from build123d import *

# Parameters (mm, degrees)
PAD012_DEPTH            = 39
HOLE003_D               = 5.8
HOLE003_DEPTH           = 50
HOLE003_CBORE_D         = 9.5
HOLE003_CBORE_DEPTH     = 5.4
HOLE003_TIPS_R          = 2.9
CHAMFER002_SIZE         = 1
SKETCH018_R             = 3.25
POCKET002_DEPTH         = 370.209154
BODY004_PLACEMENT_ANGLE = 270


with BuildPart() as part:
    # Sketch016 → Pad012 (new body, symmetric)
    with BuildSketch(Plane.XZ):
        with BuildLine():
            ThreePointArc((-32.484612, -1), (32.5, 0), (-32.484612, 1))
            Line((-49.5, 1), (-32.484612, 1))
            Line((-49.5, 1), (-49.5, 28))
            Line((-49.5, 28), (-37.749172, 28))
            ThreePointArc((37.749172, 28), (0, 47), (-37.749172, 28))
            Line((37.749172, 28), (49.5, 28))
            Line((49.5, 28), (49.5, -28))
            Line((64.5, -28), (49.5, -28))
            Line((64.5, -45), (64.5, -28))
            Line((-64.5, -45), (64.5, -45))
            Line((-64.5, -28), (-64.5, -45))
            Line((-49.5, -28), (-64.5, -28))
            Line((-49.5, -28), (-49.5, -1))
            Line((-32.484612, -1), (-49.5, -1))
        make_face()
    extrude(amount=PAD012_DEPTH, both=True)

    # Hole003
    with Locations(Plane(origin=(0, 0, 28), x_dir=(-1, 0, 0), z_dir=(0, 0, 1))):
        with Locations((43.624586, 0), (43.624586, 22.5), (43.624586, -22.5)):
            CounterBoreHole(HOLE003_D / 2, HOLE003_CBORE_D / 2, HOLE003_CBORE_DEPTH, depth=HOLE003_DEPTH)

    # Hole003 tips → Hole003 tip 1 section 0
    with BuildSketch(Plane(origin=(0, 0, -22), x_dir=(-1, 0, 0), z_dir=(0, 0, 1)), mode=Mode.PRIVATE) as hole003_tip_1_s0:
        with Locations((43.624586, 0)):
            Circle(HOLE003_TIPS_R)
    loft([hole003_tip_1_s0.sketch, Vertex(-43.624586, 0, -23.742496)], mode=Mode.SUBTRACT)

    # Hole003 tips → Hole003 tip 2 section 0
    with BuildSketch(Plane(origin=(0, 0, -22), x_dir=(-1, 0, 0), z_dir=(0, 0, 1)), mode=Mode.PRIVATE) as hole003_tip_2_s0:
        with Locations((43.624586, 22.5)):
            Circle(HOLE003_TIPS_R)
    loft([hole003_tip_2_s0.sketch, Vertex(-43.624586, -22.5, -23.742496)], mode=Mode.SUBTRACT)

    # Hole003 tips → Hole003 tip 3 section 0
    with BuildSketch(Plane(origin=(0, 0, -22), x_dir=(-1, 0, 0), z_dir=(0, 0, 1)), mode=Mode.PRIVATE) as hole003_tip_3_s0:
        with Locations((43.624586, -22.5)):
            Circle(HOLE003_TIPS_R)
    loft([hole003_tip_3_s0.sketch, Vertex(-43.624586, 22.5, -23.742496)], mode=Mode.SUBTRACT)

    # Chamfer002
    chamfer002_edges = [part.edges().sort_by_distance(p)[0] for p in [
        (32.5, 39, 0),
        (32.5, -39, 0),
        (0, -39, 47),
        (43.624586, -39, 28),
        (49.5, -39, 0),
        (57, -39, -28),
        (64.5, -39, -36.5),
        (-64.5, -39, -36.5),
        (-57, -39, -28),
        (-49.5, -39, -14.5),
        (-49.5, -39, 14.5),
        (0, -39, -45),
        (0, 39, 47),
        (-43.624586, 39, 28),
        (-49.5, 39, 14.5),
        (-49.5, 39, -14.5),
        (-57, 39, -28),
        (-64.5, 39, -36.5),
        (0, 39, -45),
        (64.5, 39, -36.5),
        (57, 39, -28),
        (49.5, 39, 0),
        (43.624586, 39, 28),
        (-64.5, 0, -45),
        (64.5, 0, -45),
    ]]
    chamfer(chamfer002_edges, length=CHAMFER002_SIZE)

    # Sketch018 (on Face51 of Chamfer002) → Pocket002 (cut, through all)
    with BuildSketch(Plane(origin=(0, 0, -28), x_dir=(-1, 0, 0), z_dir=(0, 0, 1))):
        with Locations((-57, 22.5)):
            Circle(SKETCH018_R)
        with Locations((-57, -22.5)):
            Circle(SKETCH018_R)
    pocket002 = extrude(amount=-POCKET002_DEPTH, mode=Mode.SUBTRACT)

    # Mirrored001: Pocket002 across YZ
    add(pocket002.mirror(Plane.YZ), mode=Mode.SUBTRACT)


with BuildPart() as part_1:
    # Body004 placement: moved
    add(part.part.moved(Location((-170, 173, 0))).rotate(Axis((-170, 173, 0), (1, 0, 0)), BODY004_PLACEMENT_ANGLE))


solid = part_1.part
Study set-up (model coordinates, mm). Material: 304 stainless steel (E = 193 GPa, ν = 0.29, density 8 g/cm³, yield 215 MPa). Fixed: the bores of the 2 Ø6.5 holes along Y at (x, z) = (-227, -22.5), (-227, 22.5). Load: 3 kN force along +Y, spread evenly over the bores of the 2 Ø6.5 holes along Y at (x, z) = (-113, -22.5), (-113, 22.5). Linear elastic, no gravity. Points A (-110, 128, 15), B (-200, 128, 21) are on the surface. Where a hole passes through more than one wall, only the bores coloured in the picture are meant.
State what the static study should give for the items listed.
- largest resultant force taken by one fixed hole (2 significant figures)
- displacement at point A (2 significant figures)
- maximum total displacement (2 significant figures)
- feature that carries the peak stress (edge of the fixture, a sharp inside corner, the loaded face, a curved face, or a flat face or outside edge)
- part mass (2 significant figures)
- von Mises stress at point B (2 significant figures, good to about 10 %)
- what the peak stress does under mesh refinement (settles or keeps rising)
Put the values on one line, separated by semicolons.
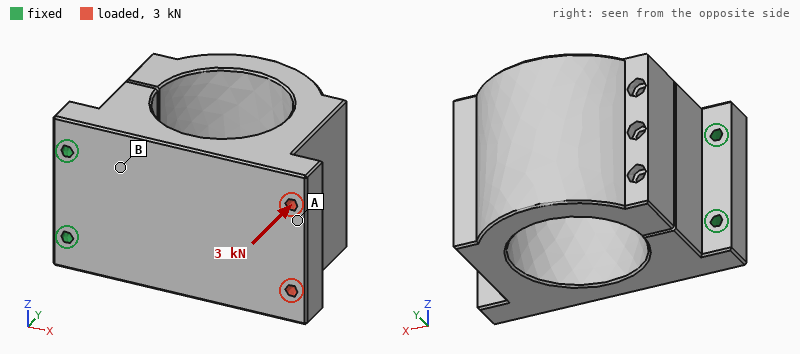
1.6 kN; 0.28 mm; 0.33 mm; edge of the fixture; 3.3 kg; 42 MPa; keeps rising
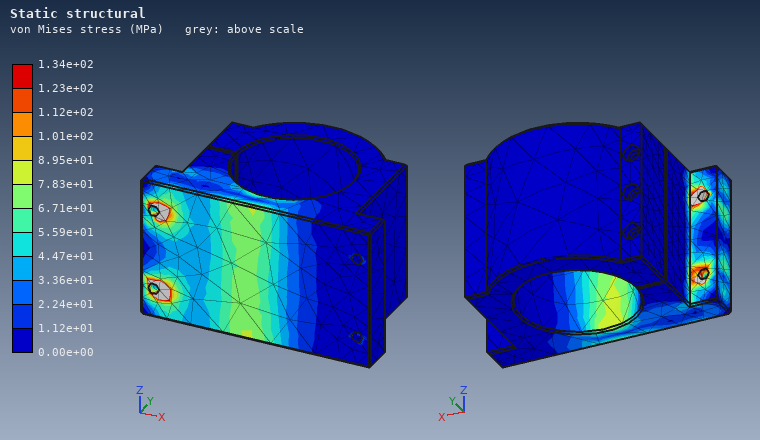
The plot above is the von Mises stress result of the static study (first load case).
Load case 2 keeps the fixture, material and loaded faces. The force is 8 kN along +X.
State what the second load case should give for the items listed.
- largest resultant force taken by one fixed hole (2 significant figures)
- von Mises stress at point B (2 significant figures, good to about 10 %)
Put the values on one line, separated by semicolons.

4.0 kN; 7.9 MPa
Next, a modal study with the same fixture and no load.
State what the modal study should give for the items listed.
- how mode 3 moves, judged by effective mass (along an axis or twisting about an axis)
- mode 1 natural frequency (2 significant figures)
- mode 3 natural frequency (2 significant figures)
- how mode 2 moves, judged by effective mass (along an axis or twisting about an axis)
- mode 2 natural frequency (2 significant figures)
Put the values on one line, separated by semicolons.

along Y; 390 Hz; 710 Hz; along Z; 660 Hz
